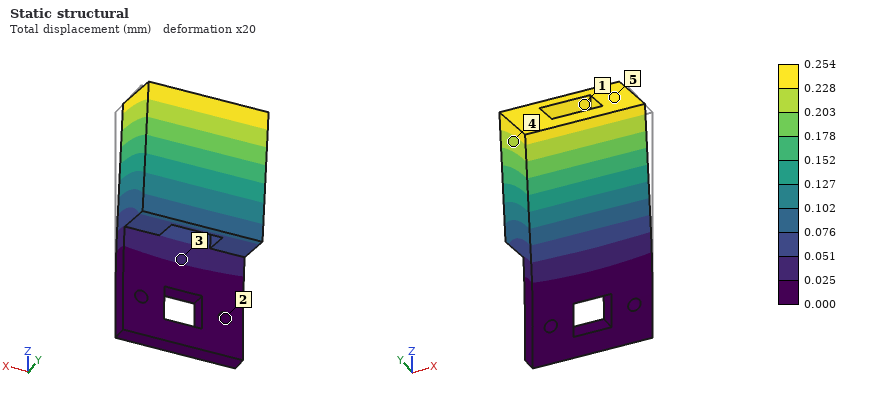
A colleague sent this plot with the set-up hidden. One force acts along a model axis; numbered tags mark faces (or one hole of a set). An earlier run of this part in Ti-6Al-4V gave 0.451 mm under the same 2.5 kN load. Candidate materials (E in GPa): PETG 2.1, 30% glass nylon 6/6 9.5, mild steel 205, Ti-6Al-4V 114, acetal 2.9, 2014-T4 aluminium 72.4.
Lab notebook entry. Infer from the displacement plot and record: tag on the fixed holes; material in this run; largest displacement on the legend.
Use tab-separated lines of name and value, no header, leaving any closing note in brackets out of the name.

tag on the fixed holes	2
material in this run	mild steel
largest displacement on the legend	0.254 mm
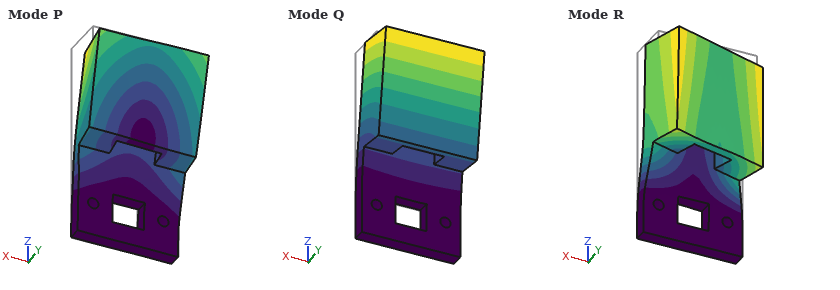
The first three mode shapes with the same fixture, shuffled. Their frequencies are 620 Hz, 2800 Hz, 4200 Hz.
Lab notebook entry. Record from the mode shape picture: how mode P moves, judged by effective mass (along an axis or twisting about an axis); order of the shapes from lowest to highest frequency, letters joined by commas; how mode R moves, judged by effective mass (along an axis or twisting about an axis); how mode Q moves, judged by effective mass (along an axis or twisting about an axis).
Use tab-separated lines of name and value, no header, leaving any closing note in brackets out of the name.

how mode P moves, judged by effective mass	along X
order of the shapes from lowest to highest frequency, letters joined by commas	Q, R, P
how mode R moves, judged by effective mass	along X
how mode Q moves, judged by effective mass	along Y
